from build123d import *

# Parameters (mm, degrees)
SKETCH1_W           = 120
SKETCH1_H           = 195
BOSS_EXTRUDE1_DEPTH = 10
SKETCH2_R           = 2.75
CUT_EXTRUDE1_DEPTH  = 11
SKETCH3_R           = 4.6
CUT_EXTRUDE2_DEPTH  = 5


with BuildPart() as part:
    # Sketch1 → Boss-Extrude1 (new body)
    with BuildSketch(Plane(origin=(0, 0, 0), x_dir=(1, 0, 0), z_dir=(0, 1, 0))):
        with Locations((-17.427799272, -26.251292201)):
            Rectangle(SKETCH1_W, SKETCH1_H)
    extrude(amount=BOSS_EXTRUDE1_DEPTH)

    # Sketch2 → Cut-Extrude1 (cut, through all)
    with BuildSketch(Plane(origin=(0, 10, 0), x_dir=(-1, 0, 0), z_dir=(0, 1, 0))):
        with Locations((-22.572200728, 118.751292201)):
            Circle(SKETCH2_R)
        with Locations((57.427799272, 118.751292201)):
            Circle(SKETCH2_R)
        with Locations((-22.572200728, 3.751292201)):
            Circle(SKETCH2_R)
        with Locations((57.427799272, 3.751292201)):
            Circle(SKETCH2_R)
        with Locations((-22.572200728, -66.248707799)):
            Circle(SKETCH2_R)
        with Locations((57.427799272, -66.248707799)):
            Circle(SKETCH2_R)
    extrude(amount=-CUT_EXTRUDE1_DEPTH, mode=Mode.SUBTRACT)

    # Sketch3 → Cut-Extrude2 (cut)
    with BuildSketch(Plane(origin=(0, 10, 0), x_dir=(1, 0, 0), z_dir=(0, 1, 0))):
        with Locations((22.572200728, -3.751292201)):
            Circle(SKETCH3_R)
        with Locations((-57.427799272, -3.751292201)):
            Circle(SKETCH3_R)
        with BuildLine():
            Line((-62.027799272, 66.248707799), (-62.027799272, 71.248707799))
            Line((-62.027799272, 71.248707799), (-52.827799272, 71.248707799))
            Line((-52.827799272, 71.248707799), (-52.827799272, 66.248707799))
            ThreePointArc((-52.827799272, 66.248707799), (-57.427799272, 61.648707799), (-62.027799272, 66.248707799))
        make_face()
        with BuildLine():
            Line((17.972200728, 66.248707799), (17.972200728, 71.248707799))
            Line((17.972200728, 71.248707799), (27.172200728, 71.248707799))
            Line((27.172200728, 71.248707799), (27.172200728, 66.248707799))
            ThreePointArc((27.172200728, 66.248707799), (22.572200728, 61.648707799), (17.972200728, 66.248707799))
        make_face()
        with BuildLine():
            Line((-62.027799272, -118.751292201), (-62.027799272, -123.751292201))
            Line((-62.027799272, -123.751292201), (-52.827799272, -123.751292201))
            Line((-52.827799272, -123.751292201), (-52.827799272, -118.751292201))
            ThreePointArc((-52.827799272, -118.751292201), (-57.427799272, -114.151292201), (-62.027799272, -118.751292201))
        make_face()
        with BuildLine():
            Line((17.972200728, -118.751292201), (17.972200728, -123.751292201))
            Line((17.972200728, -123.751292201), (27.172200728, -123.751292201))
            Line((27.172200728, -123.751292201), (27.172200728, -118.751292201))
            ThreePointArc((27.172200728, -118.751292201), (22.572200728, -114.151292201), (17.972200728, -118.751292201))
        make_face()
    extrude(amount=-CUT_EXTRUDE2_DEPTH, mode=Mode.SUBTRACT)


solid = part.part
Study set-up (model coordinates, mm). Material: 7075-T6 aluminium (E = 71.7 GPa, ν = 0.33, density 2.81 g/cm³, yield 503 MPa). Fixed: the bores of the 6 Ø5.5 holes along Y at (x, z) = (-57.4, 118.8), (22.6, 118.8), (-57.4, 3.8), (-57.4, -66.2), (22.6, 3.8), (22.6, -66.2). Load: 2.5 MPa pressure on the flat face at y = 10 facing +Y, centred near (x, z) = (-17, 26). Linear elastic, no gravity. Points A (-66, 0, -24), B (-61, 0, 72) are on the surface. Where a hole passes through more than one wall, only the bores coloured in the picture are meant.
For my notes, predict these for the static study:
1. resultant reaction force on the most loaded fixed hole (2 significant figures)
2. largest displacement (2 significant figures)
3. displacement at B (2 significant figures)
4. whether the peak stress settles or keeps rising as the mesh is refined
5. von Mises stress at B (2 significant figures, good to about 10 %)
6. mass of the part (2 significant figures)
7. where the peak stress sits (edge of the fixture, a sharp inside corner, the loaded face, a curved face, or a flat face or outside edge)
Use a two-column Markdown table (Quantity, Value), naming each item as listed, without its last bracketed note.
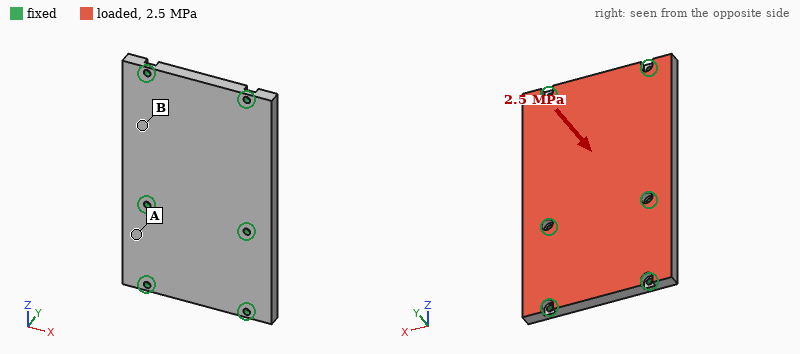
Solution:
| Quantity | Value |
|---|---|
| resultant reaction force on the most loaded fixed hole | 18 kN |
| largest displacement | 0.43 mm |
| displacement at B | 0.38 mm |
| whether the peak stress settles or keeps rising as the mesh is refined | keeps rising |
| von Mises stress at B | 110 MPa |
| mass of the part | 650 g |
| where the peak stress sits | edge of the fixture |
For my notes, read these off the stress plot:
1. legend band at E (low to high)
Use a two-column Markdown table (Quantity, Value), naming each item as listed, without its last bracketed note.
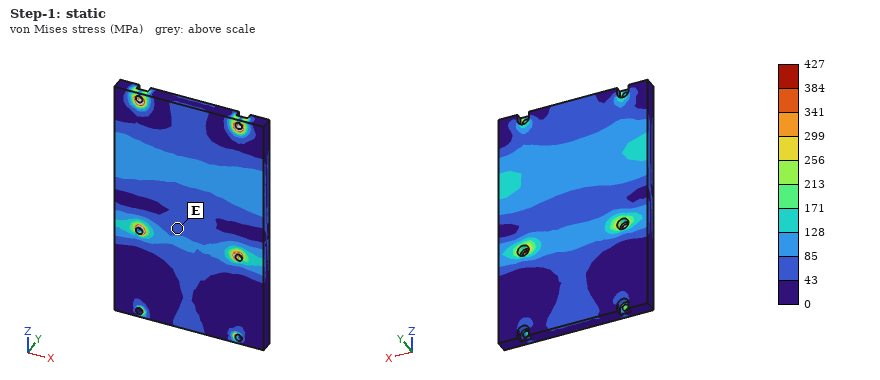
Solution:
| Quantity | Value |
|---|---|
| legend band at E | 43 to 85 MPa |
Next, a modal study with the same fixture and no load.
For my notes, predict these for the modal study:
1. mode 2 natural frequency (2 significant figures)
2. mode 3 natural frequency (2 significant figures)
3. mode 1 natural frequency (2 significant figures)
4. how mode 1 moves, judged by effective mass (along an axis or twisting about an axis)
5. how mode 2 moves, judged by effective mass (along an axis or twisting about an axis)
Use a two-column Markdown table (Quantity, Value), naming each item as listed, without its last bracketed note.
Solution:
| Quantity | Value |
|---|---|
| mode 2 natural frequency | 3400 Hz |
| mode 3 natural frequency | 4400 Hz |
| mode 1 natural frequency | 2600 Hz |
| how mode 1 moves, judged by effective mass | along Y |
| how mode 2 moves, judged by effective mass | twisting about Z |
